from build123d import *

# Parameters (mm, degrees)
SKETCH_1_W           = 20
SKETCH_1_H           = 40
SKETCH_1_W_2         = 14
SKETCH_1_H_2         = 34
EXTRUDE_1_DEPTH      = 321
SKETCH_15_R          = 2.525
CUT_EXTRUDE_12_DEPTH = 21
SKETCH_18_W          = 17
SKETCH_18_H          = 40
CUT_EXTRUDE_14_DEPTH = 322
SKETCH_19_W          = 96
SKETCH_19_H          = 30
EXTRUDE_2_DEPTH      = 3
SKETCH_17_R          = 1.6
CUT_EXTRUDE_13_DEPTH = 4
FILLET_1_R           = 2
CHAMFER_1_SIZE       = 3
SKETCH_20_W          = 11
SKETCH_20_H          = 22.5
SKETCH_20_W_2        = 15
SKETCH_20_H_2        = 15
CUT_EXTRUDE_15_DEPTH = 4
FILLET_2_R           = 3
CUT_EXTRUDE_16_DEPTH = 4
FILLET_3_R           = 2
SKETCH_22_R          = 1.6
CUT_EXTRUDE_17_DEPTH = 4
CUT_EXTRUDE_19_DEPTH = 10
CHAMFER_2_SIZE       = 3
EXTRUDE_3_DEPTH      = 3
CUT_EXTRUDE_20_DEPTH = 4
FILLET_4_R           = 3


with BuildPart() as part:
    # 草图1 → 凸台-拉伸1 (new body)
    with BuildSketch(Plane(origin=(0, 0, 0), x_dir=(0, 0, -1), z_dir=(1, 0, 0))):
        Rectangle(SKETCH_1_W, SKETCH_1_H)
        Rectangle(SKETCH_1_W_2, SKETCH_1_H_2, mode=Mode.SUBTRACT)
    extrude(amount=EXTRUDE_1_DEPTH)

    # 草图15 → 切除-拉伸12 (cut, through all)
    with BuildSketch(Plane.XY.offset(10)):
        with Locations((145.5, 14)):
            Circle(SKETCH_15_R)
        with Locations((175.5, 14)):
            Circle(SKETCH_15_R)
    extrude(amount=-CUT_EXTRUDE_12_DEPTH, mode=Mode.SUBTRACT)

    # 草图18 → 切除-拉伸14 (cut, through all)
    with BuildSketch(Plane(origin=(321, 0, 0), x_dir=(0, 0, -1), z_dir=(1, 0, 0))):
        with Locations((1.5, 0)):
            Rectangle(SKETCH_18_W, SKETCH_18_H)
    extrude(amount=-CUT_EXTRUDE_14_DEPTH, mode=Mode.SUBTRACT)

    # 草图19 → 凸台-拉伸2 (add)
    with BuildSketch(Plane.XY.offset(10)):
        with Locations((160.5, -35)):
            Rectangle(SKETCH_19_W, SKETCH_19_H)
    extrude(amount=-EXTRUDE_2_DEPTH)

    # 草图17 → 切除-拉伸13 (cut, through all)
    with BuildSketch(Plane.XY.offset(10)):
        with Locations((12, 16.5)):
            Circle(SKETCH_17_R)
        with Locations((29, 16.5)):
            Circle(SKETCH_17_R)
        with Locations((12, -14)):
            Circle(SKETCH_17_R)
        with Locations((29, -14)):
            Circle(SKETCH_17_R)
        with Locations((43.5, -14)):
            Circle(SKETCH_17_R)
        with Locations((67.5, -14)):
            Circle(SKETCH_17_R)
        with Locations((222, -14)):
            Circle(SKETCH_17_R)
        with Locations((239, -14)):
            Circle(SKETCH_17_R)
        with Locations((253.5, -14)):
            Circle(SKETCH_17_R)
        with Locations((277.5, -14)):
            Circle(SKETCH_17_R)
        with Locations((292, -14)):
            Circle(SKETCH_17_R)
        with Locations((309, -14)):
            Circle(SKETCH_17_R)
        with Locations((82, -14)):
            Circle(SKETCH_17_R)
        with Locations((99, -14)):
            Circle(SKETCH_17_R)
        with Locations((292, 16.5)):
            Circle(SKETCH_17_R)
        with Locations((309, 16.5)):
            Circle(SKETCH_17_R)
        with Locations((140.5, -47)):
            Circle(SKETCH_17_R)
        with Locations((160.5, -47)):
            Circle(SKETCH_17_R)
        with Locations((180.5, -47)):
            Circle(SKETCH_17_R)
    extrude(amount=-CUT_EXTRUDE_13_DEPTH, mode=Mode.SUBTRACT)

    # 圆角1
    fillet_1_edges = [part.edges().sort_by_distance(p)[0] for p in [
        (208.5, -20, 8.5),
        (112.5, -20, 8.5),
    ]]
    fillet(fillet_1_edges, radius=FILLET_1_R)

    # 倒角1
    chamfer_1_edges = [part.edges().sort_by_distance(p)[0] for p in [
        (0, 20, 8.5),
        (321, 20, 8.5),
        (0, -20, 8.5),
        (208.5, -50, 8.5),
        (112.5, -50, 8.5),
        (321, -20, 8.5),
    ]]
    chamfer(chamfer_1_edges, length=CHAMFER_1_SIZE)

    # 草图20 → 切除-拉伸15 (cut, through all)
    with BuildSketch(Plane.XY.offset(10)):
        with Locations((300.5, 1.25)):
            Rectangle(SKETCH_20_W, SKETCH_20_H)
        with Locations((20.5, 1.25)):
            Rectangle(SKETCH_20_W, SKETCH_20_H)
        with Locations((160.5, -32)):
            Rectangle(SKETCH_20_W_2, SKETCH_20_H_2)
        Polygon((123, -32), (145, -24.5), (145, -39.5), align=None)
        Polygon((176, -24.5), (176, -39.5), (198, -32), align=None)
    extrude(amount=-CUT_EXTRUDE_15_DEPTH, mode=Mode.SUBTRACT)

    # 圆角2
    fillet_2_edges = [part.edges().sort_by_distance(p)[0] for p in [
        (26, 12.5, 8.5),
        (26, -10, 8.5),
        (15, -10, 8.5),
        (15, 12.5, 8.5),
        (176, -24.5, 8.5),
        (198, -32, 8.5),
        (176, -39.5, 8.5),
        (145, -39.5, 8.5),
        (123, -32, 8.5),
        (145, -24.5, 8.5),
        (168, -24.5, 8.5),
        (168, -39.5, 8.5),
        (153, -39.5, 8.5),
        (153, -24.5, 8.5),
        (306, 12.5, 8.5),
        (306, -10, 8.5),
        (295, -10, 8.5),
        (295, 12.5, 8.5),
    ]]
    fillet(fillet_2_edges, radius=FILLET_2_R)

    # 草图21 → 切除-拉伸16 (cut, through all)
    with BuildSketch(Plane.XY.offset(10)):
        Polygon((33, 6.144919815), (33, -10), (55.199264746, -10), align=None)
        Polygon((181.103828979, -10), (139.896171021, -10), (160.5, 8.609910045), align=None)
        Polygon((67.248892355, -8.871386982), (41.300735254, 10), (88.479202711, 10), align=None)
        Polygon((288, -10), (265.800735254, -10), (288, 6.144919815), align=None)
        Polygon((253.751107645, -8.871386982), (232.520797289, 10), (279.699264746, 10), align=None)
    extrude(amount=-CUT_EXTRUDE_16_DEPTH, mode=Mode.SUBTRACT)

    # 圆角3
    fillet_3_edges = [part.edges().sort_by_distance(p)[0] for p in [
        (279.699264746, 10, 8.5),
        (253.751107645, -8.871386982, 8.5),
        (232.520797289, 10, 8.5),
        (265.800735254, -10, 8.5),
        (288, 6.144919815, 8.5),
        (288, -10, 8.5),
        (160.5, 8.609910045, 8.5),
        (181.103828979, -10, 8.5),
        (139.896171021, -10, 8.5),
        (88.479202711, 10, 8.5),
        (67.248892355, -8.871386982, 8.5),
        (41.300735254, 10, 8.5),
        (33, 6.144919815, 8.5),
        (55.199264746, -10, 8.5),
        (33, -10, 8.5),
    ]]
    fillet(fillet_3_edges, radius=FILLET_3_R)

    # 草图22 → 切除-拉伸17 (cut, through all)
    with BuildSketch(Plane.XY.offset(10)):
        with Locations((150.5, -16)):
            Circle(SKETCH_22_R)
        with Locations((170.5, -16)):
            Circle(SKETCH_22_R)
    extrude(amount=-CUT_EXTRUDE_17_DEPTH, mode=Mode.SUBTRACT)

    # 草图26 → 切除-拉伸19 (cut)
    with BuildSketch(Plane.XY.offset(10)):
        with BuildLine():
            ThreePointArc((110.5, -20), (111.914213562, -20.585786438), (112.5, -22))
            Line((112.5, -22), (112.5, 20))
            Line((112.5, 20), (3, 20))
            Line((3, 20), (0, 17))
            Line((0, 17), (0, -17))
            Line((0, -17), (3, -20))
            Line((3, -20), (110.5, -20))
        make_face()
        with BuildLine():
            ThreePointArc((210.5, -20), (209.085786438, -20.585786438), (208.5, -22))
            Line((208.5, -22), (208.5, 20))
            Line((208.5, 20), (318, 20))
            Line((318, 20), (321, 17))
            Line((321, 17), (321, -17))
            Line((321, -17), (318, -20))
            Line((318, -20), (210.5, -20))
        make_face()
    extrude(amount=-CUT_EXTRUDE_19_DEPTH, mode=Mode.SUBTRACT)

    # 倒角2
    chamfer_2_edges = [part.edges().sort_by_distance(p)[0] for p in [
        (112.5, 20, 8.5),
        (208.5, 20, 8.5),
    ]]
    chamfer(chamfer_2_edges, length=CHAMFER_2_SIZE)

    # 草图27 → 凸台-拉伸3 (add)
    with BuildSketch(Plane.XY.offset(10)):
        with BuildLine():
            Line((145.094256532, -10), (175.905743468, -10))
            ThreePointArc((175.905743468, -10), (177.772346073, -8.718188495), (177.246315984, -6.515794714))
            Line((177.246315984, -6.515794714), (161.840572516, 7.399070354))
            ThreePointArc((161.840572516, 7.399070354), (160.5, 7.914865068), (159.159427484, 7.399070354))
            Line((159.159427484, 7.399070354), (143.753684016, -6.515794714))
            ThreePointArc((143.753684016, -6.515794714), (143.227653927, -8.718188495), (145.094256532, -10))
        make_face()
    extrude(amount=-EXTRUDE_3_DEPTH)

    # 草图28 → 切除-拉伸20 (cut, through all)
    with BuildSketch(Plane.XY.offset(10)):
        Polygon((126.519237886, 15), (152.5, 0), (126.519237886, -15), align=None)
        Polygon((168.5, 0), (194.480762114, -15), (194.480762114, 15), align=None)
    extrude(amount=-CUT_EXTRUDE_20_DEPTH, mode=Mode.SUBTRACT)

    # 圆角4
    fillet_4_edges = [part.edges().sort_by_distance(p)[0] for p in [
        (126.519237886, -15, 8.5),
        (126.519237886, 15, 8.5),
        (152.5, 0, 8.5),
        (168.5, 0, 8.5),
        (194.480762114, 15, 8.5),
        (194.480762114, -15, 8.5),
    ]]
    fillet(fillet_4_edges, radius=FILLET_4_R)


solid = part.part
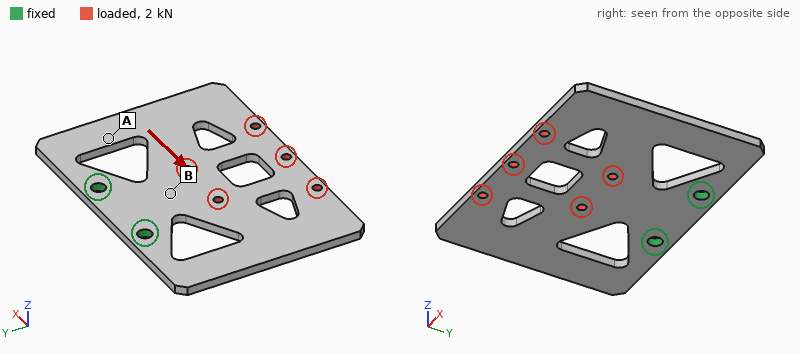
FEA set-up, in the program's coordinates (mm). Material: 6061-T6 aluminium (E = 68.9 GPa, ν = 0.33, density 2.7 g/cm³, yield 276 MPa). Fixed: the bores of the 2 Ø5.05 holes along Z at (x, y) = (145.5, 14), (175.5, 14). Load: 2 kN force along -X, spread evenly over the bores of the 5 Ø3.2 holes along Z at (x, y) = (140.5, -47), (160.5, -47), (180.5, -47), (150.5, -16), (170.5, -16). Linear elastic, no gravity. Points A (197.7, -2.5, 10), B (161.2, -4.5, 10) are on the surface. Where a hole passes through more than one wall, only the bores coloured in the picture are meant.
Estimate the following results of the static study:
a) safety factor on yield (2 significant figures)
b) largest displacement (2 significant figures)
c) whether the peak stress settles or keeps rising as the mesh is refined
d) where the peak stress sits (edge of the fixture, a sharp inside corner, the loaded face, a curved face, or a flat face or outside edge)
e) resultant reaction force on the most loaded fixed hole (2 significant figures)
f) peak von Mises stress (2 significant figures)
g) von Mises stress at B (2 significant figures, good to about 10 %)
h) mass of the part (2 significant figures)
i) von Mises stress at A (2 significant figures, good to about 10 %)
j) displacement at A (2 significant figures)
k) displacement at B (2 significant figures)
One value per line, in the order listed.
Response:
1.1
0.21 mm
settles
a curved face
3.0 kN
260 MPa
76 MPa
44 g
25 MPa
0.10 mm
0.035 mm
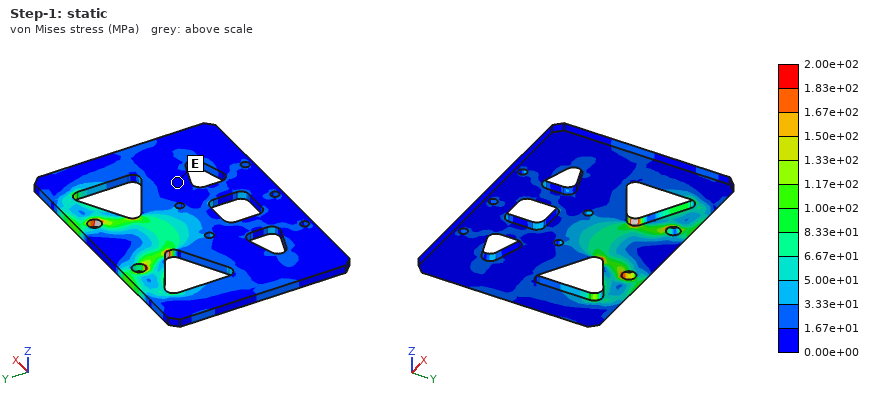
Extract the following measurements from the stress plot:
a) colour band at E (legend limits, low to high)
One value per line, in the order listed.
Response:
0.00e+00 to 1.67e+01 MPa
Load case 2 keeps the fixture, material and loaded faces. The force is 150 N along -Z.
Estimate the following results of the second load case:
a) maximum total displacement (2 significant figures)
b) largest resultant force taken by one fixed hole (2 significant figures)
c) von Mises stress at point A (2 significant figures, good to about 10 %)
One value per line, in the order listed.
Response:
1.3 mm
75 N
41 MPa
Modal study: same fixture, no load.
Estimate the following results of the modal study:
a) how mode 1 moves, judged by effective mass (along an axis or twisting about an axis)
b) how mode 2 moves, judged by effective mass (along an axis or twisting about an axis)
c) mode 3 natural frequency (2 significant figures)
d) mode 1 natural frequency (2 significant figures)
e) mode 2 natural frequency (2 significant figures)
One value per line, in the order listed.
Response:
along Z
twisting about Y
1500 Hz
430 Hz
650 Hz
